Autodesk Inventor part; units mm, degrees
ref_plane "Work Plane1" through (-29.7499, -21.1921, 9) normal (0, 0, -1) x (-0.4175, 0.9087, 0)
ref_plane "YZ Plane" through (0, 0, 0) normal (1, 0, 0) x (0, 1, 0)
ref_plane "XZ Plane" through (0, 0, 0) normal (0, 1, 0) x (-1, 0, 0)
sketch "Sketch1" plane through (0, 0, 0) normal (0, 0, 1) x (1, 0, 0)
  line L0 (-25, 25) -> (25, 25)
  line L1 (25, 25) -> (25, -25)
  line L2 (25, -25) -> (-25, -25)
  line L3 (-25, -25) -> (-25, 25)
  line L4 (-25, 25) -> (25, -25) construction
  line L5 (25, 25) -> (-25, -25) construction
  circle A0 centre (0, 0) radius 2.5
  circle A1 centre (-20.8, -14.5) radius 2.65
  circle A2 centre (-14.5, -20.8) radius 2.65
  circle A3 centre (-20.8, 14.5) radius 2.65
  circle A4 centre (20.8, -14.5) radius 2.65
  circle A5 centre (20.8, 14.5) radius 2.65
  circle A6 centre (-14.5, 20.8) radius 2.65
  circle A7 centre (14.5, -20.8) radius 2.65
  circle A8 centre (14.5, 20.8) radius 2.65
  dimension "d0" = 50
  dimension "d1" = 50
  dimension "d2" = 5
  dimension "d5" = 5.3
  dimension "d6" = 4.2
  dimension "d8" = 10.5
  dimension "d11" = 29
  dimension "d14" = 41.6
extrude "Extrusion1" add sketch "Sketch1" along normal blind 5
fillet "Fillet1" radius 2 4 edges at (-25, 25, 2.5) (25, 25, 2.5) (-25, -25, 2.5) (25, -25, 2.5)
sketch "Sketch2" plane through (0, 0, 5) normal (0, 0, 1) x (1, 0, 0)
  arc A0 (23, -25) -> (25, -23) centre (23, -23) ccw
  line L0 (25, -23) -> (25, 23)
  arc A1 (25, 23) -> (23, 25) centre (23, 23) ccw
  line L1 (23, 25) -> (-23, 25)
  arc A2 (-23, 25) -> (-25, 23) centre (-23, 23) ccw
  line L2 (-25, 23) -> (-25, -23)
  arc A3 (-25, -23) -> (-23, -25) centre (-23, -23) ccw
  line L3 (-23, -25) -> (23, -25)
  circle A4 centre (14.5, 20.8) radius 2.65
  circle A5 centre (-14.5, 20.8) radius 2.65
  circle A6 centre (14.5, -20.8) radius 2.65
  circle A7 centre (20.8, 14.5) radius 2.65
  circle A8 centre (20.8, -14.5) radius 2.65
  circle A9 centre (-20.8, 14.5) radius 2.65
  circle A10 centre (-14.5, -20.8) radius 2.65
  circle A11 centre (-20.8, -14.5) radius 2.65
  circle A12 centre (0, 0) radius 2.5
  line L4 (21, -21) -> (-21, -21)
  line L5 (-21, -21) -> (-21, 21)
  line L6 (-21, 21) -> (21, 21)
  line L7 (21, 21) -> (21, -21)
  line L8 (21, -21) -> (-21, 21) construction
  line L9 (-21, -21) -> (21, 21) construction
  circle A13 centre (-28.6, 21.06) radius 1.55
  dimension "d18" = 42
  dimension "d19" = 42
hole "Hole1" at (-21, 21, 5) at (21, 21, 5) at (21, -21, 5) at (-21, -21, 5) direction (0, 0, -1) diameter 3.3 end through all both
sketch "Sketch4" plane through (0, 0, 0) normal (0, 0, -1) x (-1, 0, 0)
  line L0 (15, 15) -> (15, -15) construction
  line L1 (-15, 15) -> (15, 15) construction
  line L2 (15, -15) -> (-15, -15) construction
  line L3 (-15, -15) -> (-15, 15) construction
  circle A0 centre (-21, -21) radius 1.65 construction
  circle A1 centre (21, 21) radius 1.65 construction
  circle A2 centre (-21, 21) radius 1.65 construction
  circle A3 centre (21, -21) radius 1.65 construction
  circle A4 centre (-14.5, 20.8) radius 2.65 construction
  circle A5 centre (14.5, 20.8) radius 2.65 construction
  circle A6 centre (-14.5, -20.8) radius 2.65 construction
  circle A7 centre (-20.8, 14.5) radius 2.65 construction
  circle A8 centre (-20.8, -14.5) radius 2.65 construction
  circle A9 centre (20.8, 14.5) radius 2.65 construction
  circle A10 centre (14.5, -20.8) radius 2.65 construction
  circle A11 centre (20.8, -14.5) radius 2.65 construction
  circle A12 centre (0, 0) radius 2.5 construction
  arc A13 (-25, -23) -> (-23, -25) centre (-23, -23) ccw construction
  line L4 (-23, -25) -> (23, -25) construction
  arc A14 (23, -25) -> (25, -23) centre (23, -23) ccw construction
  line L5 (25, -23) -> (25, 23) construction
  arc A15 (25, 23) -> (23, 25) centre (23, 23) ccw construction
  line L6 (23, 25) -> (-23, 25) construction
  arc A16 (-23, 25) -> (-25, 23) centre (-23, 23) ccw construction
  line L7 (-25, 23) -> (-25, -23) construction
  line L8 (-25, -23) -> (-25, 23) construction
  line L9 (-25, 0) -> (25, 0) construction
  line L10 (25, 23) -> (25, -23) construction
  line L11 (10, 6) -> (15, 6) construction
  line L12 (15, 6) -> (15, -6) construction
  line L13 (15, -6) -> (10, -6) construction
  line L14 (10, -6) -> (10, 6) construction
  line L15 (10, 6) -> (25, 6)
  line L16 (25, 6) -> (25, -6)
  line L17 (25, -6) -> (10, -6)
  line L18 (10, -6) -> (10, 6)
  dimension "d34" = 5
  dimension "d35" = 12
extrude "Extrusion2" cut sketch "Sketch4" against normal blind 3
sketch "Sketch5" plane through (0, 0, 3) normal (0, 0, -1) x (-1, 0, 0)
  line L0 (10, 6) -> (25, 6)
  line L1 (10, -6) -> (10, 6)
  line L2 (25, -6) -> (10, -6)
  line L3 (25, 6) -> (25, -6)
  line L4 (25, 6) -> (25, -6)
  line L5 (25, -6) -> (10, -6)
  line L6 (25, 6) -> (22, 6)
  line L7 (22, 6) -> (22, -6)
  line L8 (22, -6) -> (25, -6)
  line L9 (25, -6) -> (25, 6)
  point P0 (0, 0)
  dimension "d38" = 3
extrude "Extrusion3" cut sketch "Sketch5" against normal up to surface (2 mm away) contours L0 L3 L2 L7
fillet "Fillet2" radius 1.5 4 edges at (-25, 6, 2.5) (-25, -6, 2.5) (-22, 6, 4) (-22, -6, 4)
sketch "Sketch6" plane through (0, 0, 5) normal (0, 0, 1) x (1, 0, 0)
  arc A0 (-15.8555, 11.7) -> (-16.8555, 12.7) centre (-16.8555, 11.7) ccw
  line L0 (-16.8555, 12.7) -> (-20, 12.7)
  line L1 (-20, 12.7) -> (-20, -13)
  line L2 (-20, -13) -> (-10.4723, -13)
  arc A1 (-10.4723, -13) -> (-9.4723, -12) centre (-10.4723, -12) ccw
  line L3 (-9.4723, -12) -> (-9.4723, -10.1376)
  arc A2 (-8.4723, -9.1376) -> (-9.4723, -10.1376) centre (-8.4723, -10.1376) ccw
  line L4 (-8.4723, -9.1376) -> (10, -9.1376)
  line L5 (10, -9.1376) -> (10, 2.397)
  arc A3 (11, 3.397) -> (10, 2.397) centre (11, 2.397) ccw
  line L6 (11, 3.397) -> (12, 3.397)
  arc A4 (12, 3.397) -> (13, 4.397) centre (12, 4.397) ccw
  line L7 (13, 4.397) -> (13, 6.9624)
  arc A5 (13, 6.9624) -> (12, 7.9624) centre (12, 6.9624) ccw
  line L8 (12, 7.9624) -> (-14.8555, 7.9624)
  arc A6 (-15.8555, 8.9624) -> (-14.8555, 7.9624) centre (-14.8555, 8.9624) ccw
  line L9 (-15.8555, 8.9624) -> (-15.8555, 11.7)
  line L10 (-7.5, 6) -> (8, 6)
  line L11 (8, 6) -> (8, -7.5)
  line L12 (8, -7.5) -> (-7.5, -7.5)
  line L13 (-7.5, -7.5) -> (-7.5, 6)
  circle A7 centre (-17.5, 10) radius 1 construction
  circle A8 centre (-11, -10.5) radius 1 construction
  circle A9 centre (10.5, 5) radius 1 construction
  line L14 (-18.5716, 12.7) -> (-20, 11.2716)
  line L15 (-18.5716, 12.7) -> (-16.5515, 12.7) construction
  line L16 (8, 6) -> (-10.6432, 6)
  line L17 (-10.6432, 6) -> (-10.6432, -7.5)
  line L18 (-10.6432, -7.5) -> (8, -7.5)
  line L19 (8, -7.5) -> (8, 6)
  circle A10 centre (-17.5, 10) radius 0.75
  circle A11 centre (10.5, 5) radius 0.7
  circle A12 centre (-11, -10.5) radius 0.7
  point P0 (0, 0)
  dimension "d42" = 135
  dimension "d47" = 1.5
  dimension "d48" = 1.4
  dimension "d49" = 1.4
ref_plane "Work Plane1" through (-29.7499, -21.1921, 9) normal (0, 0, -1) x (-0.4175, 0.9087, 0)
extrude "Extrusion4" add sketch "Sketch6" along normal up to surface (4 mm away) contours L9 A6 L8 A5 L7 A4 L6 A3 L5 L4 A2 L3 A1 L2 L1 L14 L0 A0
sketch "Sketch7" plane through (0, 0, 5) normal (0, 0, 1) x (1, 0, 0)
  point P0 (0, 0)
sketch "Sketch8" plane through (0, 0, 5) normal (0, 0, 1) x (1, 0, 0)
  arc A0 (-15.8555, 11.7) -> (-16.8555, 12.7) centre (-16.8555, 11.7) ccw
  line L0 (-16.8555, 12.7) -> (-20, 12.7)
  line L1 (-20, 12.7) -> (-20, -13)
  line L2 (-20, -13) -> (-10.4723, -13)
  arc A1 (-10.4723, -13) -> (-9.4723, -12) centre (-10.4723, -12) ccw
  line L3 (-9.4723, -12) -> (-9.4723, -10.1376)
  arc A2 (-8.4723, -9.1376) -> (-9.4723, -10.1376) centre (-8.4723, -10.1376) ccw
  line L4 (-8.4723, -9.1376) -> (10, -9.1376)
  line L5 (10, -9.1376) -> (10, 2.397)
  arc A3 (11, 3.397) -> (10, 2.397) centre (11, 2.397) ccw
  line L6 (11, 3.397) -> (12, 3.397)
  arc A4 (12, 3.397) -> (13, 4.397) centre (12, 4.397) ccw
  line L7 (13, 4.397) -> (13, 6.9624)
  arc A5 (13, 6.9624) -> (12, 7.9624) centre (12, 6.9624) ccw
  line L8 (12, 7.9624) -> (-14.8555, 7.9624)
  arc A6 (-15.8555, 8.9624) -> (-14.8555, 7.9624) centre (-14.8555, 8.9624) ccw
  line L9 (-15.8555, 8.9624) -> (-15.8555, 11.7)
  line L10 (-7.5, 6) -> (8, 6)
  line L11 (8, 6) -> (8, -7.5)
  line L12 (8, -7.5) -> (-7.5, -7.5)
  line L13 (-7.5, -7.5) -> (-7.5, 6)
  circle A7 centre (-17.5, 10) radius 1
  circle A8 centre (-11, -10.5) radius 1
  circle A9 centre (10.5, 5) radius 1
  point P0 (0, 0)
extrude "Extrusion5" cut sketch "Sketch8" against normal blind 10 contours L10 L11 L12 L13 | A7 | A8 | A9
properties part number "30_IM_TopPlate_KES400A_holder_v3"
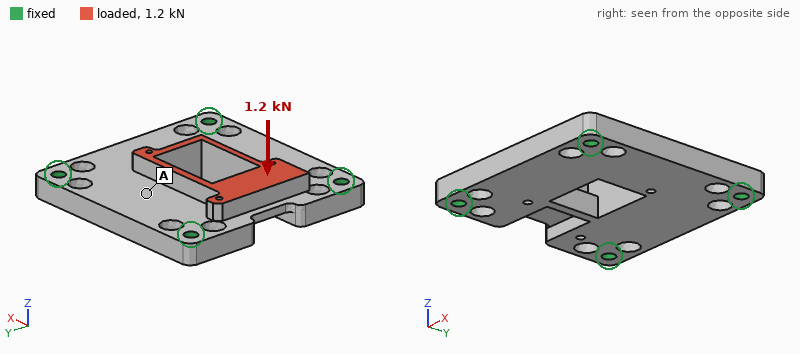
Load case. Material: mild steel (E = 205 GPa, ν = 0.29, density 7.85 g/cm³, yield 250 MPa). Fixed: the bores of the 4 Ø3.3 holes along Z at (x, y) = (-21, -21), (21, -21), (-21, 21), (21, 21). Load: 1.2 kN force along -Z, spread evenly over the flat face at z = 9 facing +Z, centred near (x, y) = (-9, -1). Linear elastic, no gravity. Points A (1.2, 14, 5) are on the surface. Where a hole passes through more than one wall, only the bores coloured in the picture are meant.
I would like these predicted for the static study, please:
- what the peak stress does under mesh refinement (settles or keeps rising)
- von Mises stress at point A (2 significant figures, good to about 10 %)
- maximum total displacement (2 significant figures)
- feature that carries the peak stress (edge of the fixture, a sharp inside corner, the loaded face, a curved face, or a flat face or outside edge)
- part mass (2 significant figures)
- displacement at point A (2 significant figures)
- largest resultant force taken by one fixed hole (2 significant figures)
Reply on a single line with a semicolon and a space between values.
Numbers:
keeps rising; 10 MPa; 11 µm; edge of the fixture; 87 g; 5.9 µm; 600 N
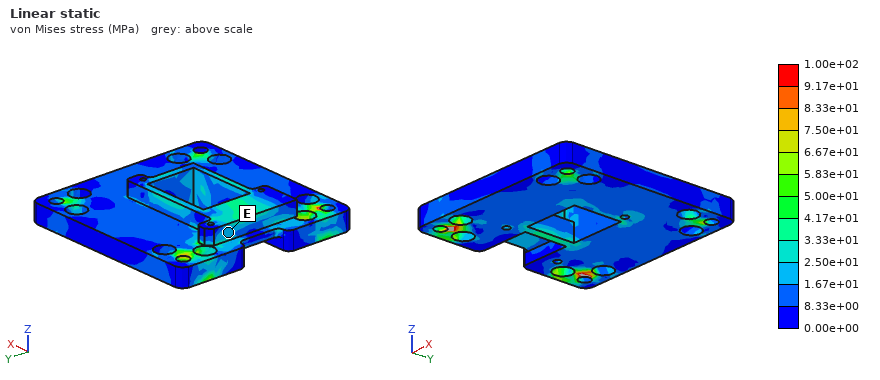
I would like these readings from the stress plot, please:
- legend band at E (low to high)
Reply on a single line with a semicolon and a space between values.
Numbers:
1.67e+01 to 2.50e+01 MPa
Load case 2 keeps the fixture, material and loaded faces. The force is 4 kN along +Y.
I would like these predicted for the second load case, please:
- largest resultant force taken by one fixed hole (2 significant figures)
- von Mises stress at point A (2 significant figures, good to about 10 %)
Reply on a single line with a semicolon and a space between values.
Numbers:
1.5 kN; 16 MPa
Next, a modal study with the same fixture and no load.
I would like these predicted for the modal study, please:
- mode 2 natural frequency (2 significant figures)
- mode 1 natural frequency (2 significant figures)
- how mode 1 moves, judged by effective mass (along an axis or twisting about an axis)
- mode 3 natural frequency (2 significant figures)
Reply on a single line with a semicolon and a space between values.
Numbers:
14 kHz; 8800 Hz; along Z; 14 kHz
